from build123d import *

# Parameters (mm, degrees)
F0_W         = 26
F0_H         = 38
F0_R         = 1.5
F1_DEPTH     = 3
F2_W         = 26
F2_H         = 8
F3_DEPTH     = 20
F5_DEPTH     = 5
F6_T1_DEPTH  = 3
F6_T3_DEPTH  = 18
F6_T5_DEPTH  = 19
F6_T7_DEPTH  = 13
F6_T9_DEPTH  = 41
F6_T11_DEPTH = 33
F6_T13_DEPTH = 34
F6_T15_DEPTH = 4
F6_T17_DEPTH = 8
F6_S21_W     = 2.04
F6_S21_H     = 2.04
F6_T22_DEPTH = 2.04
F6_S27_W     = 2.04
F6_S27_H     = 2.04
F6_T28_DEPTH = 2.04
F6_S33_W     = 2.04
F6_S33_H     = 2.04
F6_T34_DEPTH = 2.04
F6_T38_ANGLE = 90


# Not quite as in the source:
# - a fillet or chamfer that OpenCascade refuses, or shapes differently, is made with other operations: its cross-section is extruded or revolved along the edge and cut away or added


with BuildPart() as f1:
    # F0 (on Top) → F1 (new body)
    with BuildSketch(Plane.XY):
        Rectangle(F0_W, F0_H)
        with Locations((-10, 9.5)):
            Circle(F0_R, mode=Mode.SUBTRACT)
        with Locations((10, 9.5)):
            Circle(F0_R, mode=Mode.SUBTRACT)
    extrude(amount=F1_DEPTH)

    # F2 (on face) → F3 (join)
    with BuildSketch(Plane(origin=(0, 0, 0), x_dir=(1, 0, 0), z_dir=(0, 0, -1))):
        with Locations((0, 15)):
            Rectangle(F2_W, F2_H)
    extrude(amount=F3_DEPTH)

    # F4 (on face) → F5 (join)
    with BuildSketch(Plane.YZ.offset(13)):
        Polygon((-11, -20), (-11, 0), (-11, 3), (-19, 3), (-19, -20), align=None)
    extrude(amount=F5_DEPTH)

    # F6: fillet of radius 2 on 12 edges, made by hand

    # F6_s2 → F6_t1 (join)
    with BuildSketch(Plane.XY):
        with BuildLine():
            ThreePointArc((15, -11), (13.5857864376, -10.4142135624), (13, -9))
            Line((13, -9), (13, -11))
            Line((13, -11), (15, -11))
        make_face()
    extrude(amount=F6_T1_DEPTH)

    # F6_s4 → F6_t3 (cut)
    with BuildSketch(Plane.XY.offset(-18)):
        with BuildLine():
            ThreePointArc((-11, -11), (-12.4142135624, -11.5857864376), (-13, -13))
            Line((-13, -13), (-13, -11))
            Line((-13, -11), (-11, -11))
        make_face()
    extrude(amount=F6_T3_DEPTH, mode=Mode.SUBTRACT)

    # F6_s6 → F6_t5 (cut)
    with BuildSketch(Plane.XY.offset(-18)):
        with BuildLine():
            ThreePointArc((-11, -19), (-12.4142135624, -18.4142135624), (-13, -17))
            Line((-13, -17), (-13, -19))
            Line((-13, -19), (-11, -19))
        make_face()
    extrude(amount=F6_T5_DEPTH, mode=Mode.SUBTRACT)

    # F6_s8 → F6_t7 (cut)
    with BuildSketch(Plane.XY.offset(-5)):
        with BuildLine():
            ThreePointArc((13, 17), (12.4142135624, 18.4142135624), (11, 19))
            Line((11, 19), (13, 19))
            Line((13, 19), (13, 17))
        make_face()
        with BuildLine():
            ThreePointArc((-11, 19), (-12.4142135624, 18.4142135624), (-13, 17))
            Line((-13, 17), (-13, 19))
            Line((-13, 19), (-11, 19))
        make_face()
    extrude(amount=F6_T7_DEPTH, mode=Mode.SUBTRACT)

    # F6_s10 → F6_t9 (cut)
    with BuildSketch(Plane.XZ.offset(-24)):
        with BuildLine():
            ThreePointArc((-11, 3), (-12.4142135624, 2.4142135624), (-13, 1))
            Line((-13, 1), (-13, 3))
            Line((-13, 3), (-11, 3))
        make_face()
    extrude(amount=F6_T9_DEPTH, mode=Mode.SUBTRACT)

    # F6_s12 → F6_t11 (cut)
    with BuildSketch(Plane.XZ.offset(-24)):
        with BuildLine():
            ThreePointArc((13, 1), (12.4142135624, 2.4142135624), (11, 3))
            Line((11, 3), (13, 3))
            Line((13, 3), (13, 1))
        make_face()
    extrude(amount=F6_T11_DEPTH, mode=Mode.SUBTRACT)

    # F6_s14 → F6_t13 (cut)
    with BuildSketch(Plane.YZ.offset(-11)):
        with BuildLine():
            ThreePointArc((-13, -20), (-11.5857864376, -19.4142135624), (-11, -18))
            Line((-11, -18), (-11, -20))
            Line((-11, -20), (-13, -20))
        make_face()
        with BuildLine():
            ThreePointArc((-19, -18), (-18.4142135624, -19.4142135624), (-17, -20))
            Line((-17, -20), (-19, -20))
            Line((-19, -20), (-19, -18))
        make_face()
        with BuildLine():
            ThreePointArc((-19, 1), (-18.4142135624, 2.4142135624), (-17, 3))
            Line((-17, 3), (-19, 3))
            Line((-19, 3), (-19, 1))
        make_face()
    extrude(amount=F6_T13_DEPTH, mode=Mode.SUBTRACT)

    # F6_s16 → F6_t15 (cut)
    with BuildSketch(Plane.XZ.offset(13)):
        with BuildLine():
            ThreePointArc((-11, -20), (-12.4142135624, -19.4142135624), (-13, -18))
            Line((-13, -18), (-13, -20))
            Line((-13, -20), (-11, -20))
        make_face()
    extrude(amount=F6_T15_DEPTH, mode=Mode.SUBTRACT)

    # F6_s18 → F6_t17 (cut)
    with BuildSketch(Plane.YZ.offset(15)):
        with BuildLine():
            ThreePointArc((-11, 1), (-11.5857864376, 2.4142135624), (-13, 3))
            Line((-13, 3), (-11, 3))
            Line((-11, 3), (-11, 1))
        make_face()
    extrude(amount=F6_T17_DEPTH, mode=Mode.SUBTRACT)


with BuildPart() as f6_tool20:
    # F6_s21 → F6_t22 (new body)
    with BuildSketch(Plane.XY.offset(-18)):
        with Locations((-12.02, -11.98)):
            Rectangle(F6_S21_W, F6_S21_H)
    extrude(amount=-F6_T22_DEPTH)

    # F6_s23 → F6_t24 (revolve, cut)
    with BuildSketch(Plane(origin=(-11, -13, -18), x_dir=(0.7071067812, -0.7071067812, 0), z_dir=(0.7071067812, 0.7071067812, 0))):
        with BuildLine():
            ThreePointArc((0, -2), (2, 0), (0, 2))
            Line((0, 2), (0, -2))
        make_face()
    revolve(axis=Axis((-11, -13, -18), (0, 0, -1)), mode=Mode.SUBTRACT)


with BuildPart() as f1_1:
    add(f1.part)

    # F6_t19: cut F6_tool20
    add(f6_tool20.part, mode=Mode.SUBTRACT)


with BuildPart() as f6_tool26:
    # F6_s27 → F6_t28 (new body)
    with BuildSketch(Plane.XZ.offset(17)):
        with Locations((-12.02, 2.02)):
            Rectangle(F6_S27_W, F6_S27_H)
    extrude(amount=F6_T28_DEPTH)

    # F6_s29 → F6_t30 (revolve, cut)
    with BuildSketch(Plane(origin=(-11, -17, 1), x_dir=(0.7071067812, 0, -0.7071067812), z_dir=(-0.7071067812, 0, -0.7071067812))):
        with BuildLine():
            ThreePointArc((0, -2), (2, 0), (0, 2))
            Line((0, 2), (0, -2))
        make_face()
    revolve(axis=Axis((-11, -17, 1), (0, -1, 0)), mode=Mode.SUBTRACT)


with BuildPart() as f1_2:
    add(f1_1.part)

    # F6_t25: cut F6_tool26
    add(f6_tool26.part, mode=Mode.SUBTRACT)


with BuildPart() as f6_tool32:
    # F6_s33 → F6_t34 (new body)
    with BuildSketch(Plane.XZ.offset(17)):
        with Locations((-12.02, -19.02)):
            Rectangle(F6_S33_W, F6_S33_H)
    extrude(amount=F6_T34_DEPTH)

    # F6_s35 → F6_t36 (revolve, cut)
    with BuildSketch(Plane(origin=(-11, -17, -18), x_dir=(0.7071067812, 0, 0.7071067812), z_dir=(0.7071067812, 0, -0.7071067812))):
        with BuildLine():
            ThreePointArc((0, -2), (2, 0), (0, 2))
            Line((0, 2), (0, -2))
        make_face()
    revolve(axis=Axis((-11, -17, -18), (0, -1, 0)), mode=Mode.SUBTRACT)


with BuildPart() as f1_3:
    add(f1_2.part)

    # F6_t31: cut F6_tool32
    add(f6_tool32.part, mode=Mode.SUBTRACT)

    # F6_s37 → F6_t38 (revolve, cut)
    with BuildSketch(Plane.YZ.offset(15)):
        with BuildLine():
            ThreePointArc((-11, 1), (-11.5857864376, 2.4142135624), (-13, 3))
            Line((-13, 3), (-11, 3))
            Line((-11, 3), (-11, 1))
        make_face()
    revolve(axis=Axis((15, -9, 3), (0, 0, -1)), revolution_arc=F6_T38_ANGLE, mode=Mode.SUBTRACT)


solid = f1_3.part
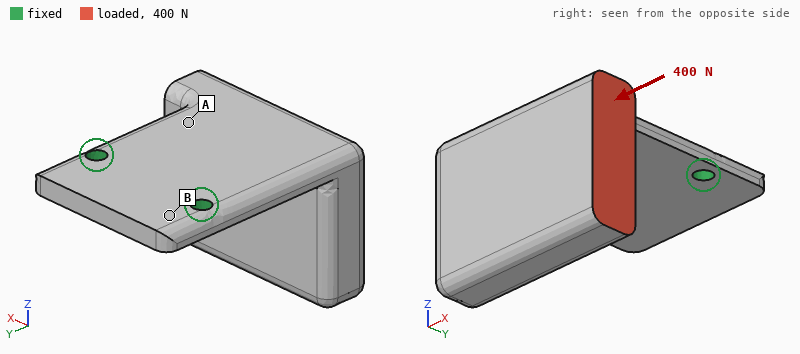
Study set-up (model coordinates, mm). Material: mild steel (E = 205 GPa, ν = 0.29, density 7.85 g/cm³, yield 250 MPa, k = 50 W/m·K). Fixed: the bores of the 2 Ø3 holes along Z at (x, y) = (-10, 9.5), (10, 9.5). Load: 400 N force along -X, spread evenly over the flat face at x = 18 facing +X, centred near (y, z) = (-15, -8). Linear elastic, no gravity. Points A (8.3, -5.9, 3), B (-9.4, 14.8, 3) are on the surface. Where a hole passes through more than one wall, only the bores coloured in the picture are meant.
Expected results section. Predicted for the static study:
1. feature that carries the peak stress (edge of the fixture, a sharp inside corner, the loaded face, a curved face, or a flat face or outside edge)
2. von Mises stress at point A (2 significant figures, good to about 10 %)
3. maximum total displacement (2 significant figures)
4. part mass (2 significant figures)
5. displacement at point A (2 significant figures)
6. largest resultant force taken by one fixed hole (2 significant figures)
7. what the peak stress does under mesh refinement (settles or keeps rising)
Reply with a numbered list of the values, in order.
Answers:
1. edge of the fixture
2. 52 MPa
3. 74 µm
4. 61 g
5. 16 µm
6. 550 N
7. keeps rising
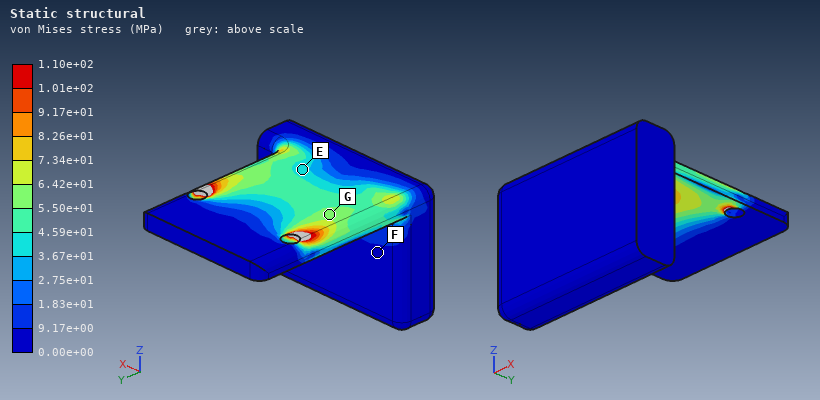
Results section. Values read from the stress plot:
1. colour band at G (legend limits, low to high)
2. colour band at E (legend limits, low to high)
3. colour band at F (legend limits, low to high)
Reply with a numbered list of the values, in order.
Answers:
1. 5.50e+01 to 6.42e+01 MPa
2. 3.67e+01 to 4.59e+01 MPa
3. 0.00e+00 to 9.17e+00 MPa
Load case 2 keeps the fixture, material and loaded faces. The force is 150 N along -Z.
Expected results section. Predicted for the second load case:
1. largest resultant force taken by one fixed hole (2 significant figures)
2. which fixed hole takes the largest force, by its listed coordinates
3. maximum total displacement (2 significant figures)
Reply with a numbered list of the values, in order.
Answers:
1. 210 N
2. (10, 9.5)
3. 0.14 mm
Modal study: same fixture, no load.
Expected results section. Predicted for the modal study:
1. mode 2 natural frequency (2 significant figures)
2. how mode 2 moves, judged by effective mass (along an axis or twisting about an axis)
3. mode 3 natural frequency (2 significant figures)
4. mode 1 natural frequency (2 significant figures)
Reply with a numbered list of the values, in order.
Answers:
1. 2000 Hz
2. along X
3. 3900 Hz
4. 910 Hz
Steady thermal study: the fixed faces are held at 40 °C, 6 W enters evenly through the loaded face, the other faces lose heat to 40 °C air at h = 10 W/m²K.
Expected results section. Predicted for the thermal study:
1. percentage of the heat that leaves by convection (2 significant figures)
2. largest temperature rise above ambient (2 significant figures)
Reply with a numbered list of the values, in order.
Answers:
1. 14 %
2. 44 K
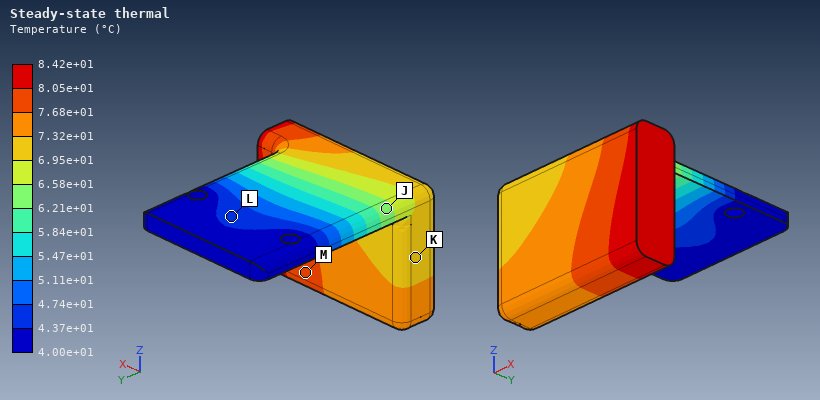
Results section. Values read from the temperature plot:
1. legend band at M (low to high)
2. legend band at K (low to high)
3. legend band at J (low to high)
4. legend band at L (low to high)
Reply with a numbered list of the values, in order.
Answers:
1. 7.68e+01 to 8.05e+01 °C
2. 6.95e+01 to 7.32e+01 °C
3. 6.21e+01 to 6.58e+01 °C
4. 4.37e+01 to 4.74e+01 °C
